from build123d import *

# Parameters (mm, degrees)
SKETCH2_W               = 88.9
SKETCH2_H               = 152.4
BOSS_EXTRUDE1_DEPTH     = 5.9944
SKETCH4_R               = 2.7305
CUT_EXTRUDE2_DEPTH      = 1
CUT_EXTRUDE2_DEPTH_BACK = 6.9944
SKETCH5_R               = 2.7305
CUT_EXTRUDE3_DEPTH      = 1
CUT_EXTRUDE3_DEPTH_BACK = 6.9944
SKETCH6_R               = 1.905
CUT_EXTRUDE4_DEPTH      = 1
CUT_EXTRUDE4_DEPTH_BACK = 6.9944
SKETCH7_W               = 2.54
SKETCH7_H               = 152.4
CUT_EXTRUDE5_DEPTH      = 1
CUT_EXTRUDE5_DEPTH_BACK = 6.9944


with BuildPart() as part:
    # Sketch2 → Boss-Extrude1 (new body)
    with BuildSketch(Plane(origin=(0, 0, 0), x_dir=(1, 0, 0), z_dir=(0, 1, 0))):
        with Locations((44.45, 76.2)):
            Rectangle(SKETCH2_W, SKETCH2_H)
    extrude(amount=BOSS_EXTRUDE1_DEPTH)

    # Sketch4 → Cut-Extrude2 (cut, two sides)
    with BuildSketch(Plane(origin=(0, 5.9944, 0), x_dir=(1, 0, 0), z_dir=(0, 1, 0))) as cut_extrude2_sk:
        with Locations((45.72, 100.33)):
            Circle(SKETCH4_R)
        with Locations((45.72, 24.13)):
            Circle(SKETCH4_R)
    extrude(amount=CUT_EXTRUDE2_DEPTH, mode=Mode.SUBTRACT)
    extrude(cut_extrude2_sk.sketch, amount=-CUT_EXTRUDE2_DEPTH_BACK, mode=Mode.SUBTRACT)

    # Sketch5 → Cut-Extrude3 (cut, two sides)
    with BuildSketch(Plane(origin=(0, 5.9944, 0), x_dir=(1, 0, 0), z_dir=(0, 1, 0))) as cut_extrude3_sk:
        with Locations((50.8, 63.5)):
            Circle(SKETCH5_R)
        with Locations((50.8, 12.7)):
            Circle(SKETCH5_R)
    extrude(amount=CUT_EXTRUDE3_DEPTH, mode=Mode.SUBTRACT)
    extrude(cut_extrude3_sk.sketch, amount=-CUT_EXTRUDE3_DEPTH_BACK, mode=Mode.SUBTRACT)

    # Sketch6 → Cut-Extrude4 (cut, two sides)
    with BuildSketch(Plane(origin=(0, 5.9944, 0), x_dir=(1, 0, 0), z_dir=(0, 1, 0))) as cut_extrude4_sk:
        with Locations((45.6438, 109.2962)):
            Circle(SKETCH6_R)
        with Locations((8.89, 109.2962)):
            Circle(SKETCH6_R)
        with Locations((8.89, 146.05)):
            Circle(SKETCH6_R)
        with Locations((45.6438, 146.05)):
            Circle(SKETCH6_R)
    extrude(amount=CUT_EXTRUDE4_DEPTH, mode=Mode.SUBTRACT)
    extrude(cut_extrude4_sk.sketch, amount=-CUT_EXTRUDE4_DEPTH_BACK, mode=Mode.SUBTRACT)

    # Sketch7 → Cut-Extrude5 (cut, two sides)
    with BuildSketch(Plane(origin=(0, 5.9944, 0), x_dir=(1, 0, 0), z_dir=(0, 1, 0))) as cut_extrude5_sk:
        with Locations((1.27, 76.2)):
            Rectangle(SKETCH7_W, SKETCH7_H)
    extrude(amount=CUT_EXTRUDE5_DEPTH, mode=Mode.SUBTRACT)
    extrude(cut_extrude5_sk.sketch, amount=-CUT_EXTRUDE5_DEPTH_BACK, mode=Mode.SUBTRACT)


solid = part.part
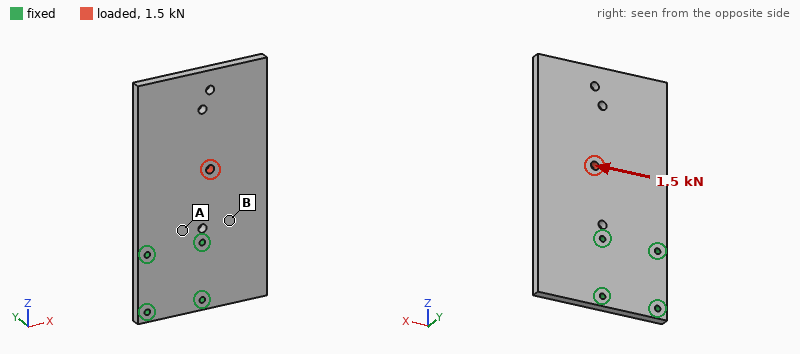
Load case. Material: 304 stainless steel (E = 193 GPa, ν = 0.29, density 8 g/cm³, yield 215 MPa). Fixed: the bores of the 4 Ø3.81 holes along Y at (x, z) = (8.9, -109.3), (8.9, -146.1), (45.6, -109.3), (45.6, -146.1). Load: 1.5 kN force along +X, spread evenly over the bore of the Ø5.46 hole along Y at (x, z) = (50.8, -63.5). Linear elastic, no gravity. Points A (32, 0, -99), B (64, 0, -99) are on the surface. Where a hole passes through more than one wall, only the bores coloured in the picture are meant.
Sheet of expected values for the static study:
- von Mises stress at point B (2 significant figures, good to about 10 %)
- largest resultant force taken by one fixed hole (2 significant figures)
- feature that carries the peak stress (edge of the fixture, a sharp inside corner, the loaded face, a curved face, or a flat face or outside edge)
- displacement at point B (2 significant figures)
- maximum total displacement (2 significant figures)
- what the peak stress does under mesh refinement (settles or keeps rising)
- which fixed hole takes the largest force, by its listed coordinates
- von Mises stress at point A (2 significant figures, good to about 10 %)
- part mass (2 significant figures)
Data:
4.7 MPa
1.6 kN
edge of the fixture
2.3 µm
9.8 µm
keeps rising
(45.6, -109.3)
9.6 MPa
620 g
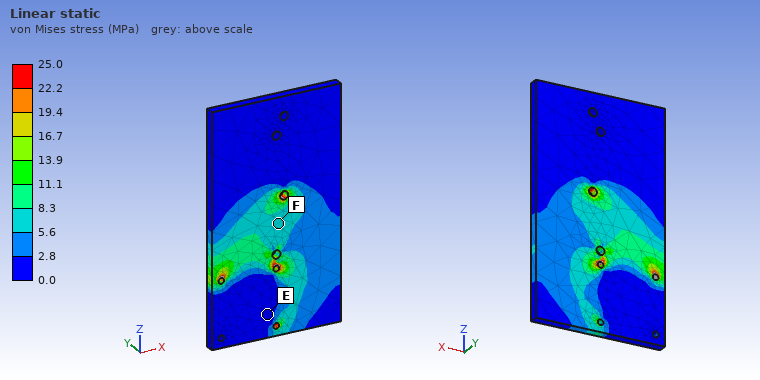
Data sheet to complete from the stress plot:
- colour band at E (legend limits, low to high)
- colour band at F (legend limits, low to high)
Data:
0.0 to 2.8 MPa
5.6 to 8.3 MPa
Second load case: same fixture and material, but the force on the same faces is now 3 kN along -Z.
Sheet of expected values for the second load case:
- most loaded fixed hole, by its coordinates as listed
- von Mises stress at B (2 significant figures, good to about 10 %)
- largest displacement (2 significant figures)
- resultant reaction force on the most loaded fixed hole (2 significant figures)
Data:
(45.6, -109.3)
7.0 MPa
7.3 µm
2.0 kN
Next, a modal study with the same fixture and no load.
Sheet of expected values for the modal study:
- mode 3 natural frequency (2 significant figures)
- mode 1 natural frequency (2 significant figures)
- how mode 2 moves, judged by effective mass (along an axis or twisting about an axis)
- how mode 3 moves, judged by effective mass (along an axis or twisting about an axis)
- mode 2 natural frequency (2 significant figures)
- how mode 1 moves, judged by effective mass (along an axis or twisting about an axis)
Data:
2100 Hz
370 Hz
twisting about Z
along Y
1000 Hz
along Y
